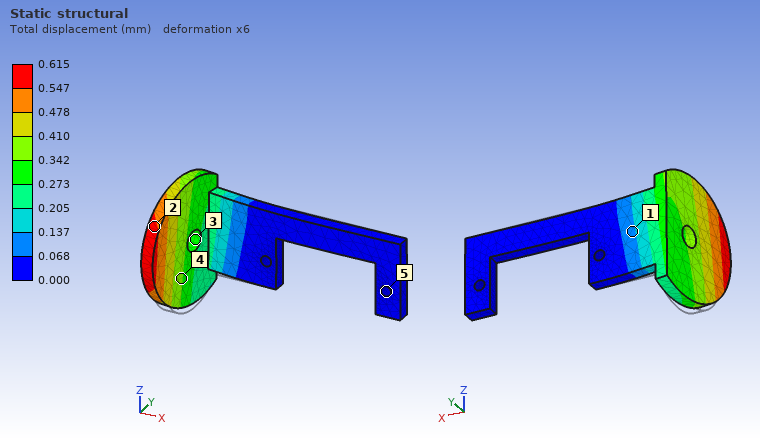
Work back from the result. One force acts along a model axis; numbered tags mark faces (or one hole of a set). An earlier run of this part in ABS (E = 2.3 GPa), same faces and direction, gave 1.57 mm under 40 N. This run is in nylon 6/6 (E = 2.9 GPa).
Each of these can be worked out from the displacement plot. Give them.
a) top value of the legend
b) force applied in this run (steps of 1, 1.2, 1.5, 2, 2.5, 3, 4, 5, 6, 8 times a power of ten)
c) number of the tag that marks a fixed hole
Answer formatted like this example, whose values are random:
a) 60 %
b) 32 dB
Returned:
a) 0.615 mm
b) 20 N
c) 5
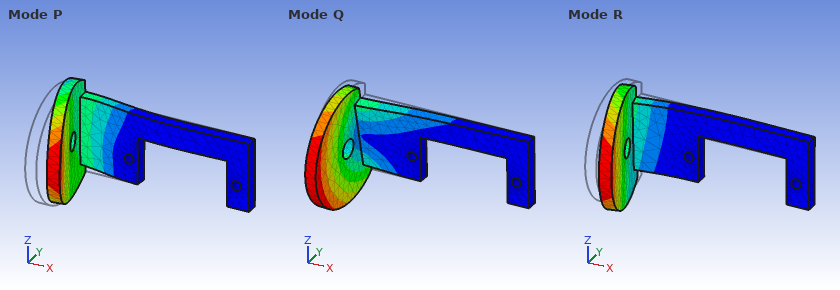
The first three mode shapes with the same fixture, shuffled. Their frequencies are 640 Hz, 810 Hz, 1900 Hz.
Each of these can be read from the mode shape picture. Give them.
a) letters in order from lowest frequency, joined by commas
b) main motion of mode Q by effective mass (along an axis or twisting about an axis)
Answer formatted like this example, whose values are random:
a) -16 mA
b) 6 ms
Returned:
a) R, Q, P
b) along Z
